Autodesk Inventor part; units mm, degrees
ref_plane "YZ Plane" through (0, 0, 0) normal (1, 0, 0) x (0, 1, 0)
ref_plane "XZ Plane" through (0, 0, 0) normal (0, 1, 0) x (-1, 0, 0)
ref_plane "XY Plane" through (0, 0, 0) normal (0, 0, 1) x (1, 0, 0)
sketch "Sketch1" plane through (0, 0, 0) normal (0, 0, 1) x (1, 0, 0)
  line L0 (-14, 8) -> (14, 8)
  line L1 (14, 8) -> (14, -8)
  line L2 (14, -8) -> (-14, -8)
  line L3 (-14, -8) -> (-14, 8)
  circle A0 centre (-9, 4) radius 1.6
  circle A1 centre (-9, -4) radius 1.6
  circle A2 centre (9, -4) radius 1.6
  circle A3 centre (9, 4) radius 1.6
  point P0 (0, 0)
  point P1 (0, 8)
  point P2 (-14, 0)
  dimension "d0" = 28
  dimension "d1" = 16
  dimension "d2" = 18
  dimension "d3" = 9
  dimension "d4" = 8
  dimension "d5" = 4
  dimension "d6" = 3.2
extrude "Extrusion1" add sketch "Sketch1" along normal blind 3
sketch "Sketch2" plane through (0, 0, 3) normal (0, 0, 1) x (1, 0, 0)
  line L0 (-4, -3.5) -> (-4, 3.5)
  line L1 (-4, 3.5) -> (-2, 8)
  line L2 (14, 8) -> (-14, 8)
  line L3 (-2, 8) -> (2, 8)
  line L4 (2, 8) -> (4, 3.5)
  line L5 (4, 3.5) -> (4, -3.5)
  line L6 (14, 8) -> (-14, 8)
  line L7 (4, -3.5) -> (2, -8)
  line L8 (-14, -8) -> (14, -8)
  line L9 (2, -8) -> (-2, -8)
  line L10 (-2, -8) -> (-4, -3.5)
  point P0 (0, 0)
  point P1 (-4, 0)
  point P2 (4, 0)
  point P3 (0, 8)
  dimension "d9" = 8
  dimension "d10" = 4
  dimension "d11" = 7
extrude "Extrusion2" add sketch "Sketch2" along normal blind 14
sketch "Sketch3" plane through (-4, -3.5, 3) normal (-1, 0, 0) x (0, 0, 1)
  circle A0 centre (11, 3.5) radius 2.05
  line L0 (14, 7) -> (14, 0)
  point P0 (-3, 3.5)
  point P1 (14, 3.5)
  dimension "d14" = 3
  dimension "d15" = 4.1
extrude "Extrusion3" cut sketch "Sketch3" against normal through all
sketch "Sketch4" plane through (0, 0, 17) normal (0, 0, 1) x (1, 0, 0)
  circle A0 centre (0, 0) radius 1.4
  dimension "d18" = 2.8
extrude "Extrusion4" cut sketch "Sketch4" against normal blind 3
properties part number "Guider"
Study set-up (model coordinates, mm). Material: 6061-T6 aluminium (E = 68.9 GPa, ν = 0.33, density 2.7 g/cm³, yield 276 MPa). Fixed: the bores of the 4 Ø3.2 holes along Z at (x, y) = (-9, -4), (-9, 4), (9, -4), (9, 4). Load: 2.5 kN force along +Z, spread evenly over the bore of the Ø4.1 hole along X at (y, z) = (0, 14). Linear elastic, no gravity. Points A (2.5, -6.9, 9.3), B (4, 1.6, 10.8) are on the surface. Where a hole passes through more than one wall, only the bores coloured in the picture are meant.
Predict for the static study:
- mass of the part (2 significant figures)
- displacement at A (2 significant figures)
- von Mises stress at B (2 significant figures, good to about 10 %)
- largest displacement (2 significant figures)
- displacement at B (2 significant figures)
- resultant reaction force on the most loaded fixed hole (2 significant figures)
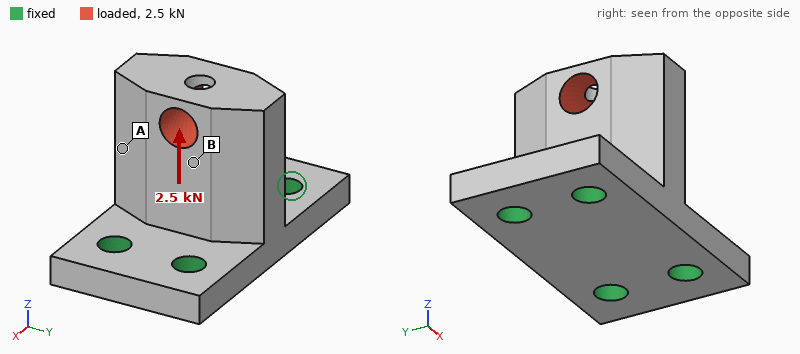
7.2 g
16 µm
39 MPa
25 µm
18 µm
660 N
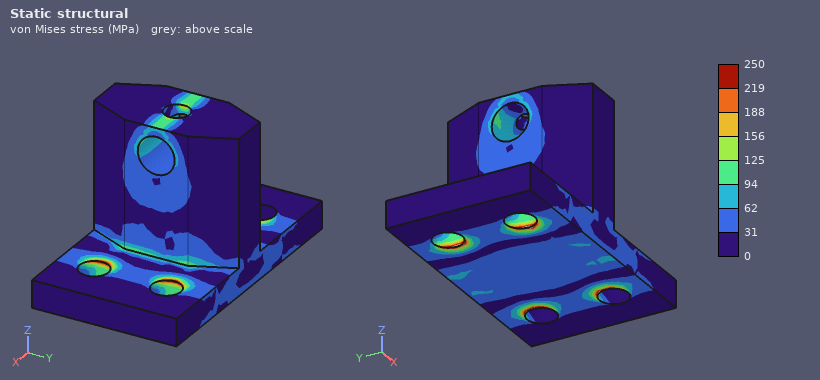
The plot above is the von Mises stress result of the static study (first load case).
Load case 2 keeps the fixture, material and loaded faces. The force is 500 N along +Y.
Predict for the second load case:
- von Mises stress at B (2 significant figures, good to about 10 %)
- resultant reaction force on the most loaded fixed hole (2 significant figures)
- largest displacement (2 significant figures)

12 MPa
340 N
35 µm
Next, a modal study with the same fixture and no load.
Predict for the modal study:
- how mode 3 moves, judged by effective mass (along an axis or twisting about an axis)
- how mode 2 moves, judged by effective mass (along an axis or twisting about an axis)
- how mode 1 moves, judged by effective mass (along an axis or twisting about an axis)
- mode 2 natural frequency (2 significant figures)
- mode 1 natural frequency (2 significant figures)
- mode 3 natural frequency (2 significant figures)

along Z
along X
along Y
17 kHz
14 kHz
28 kHz
